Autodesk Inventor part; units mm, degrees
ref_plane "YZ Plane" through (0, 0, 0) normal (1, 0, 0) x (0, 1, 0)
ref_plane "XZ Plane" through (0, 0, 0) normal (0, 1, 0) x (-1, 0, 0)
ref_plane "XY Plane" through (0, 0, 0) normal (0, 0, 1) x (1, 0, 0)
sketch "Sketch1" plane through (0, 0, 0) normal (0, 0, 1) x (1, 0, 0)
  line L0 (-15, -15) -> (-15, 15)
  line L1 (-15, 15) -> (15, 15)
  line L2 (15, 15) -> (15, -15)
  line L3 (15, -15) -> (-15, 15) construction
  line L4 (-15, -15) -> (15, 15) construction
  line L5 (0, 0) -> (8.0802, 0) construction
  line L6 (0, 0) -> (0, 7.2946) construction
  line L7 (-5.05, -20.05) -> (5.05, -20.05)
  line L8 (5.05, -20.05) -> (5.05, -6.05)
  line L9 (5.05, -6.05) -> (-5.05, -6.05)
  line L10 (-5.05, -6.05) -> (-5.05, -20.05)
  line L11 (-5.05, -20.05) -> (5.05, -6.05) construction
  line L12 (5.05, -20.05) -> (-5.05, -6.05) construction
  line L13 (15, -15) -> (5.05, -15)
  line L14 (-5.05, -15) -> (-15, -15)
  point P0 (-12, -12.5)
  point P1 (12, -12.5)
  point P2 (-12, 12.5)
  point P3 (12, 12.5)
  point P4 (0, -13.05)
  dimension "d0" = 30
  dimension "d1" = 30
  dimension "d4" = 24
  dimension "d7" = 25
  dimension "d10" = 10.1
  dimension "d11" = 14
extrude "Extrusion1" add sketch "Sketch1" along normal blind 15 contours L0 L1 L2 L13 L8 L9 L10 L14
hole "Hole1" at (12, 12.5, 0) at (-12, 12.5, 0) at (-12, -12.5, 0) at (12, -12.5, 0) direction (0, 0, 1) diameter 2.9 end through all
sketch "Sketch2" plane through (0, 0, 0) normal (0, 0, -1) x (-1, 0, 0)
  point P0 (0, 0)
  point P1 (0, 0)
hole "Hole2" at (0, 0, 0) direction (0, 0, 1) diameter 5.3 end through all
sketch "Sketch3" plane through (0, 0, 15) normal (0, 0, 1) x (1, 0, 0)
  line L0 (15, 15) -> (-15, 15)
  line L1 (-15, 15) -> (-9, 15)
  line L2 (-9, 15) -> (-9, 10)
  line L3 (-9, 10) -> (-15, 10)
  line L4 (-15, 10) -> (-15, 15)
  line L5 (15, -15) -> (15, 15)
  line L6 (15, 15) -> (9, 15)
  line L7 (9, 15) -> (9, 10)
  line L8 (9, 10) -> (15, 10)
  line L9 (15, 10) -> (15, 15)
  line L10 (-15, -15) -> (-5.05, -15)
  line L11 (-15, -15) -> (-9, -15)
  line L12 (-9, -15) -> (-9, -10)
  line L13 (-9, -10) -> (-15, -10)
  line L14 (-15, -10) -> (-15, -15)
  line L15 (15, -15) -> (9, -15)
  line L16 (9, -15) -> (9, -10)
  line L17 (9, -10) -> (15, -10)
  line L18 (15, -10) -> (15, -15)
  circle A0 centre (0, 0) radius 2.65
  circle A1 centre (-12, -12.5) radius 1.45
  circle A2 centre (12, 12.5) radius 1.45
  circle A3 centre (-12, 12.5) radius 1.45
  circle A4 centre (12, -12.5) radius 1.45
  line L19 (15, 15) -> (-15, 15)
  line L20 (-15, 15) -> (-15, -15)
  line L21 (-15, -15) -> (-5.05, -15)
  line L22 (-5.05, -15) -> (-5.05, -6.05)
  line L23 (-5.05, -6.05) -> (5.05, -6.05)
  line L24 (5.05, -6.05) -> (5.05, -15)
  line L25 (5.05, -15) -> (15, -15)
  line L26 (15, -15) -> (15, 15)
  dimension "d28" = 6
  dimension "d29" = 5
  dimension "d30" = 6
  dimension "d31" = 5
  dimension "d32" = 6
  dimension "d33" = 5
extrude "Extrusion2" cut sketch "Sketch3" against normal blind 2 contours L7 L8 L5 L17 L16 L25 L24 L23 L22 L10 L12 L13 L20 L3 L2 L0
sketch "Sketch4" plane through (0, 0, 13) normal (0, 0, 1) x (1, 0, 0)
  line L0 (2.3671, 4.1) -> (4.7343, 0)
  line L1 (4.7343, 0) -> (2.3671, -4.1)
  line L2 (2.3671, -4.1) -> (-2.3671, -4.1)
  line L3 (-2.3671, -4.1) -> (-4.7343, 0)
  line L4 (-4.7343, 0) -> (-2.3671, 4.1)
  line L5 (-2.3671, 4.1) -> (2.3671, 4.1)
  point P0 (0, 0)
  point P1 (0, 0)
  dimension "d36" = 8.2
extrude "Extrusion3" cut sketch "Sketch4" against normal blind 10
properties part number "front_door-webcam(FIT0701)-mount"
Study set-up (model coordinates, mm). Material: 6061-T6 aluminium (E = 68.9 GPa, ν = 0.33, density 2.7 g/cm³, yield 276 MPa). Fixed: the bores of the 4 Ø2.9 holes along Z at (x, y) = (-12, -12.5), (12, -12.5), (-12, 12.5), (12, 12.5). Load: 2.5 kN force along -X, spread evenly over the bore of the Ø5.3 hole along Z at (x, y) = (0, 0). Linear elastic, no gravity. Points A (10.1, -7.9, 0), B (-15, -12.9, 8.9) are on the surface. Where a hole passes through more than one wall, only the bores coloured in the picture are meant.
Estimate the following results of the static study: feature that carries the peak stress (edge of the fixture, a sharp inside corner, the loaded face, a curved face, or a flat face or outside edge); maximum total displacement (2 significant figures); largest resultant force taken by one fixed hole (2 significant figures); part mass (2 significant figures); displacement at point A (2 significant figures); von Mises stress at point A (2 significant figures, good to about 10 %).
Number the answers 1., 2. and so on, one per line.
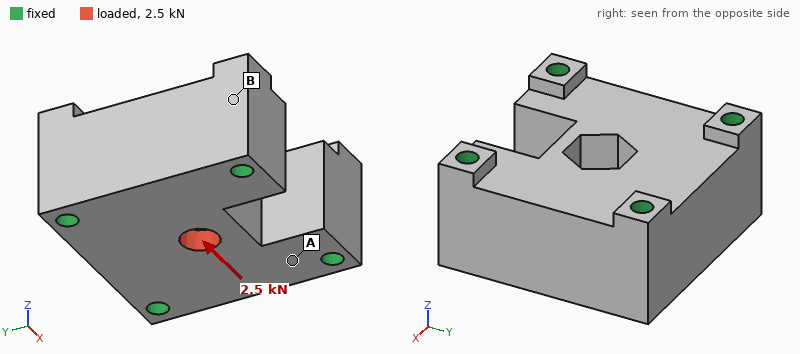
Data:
1. a sharp inside corner
2. 6.6 µm
3. 980 N
4. 26 g
5. 1.7 µm
6. 17 MPa
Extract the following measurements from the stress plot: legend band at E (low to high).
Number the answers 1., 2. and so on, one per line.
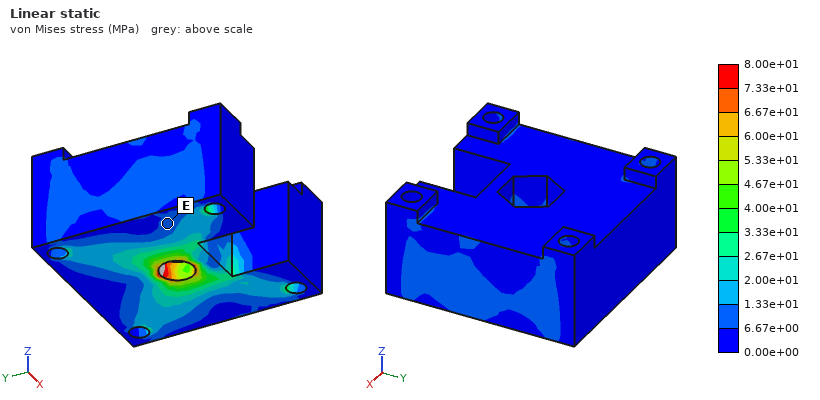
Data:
1. 6.67e+00 to 1.33e+01 MPa
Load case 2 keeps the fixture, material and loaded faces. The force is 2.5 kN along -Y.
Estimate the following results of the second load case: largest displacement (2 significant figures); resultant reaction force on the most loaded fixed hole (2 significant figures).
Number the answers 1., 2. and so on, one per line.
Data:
1. 9.9 µm
2. 810 N
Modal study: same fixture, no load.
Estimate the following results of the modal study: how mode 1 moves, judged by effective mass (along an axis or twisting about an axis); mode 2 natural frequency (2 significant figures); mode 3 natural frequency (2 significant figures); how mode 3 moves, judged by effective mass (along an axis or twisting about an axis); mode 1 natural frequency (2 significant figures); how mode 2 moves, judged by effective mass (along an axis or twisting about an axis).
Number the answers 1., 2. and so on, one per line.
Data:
1. along Z
2. 46 kHz
3. 53 kHz
4. twisting about Y
5. 42 kHz
6. along X
